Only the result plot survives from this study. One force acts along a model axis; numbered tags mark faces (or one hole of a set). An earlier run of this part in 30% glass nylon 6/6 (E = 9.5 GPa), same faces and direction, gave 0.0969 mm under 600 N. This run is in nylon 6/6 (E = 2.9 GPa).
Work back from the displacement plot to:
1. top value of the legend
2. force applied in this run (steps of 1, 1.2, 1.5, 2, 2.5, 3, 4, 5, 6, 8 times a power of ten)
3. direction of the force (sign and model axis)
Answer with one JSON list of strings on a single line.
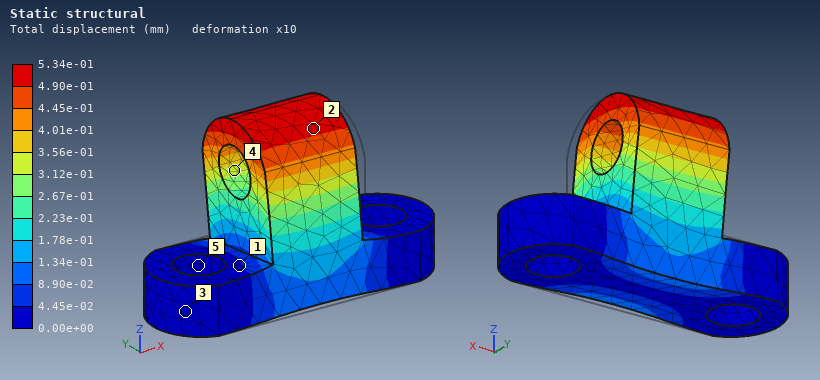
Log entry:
["5.34e-01 mm", "1 kN", "+Y"]
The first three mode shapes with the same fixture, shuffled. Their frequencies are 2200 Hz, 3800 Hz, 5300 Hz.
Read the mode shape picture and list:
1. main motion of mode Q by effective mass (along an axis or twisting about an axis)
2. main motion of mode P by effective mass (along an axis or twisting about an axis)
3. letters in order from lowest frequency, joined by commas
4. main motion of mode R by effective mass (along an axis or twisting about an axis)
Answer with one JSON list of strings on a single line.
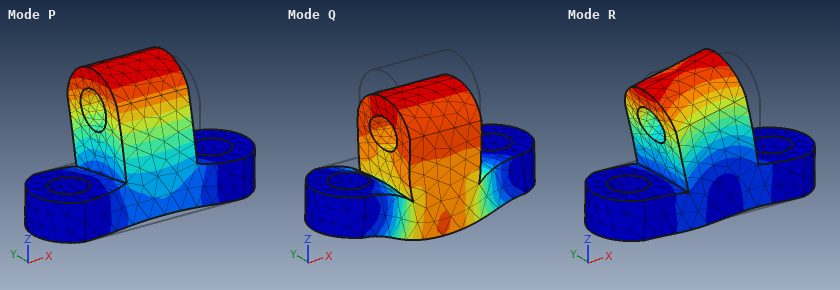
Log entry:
["along Z", "along Y", "P, R, Q", "along X"]
